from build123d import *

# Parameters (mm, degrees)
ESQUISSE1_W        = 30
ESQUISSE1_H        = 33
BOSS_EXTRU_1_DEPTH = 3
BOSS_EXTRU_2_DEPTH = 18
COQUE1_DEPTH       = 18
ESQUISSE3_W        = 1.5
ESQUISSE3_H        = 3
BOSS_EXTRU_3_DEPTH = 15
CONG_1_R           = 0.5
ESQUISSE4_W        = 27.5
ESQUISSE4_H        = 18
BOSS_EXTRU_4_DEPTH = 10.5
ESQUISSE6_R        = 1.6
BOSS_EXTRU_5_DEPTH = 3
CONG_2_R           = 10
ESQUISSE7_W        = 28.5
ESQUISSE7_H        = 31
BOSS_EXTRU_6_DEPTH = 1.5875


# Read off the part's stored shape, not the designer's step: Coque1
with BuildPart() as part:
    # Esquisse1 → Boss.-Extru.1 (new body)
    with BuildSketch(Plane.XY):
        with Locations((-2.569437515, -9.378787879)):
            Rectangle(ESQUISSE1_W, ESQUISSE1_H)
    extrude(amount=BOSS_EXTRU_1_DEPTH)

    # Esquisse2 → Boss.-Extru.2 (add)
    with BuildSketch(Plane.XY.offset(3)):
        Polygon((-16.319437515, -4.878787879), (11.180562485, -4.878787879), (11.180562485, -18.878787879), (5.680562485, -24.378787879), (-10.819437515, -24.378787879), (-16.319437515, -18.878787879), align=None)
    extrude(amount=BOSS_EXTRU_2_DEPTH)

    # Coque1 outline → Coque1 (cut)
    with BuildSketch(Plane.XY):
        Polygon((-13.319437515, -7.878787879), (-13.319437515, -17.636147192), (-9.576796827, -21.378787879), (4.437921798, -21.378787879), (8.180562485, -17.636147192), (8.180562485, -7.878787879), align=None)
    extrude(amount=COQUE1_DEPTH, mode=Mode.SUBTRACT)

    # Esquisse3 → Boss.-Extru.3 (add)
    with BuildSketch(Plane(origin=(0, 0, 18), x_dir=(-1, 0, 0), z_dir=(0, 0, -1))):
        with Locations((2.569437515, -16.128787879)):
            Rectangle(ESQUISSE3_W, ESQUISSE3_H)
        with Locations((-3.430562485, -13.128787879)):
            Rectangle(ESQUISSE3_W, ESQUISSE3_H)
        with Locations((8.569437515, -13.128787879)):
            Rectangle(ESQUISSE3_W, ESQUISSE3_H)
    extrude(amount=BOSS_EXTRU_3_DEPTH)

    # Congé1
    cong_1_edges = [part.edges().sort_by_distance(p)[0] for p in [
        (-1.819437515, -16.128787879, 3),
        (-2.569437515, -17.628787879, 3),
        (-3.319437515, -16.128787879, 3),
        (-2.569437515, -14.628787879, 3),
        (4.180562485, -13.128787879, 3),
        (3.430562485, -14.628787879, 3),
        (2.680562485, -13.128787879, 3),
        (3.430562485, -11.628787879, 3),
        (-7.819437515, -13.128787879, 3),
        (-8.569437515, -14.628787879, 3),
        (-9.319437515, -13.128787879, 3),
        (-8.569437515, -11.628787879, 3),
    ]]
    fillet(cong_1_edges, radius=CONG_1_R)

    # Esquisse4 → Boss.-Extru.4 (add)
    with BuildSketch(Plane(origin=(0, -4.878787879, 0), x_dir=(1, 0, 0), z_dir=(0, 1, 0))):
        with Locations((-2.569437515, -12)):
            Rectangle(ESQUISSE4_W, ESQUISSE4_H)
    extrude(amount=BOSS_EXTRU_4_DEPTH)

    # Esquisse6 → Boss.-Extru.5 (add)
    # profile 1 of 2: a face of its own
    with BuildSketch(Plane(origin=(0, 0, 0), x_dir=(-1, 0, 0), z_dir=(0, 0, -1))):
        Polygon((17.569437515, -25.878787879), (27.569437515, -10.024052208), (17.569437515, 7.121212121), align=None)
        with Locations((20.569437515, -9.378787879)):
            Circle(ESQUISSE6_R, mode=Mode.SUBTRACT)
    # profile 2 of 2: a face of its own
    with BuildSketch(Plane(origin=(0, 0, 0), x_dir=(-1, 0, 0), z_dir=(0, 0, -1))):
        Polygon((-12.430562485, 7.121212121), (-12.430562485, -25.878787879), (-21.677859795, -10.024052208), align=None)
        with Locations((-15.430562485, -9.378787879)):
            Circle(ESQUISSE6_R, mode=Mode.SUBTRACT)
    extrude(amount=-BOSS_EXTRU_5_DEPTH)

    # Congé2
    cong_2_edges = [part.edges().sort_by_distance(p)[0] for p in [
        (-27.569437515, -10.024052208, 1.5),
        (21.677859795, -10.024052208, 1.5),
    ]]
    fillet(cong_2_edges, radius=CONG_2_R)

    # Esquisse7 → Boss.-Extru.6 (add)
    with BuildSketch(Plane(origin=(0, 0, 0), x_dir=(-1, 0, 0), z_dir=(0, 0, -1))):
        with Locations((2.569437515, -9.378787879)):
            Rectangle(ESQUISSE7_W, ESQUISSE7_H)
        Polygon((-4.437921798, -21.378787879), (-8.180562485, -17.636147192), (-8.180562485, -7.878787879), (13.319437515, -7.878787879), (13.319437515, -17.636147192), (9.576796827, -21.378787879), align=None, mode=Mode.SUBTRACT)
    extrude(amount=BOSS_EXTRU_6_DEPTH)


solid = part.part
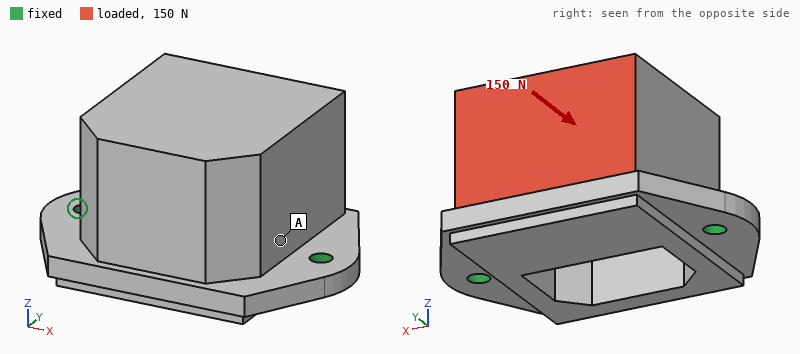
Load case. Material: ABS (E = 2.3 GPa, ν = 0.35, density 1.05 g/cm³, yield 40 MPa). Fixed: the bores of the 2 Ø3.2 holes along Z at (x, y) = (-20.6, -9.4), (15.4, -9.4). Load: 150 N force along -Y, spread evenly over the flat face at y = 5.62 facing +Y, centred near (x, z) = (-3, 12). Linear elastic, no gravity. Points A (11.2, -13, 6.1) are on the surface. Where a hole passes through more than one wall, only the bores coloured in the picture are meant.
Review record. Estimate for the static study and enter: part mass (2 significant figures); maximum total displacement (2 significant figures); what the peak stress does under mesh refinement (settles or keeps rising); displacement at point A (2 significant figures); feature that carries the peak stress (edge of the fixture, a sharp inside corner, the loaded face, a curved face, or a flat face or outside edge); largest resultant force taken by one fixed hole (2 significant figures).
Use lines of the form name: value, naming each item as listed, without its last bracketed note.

part mass: 15 g
maximum total displacement: 0.57 mm
what the peak stress does under mesh refinement: keeps rising
displacement at point A: 0.14 mm
feature that carries the peak stress: edge of the fixture
largest resultant force taken by one fixed hole: 77 N
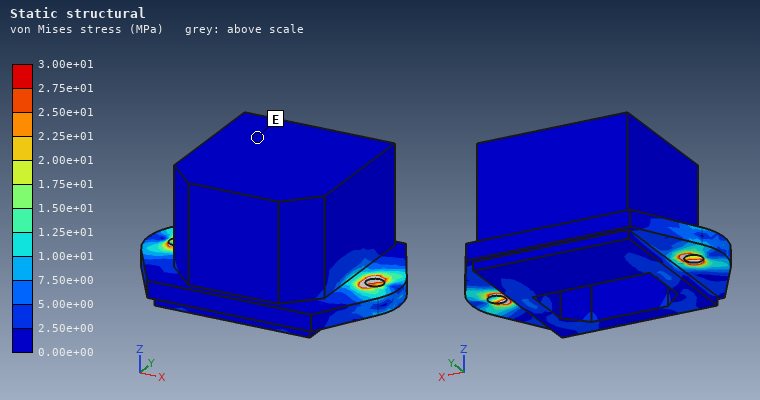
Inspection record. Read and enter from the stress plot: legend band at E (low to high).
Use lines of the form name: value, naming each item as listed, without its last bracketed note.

legend band at E: 0.00e+00 to 2.50e+00 MPa
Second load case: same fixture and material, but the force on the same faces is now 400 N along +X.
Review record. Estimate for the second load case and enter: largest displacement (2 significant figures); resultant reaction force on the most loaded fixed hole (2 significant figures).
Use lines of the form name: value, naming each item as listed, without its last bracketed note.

largest displacement: 0.14 mm
resultant reaction force on the most loaded fixed hole: 290 N
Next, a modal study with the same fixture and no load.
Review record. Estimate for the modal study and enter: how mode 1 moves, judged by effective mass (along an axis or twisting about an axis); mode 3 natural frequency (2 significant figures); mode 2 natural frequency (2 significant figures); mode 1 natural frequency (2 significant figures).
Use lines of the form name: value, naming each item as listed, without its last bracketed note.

how mode 1 moves, judged by effective mass: along Y
mode 3 natural frequency: 1600 Hz
mode 2 natural frequency: 1600 Hz
mode 1 natural frequency: 770 Hz
